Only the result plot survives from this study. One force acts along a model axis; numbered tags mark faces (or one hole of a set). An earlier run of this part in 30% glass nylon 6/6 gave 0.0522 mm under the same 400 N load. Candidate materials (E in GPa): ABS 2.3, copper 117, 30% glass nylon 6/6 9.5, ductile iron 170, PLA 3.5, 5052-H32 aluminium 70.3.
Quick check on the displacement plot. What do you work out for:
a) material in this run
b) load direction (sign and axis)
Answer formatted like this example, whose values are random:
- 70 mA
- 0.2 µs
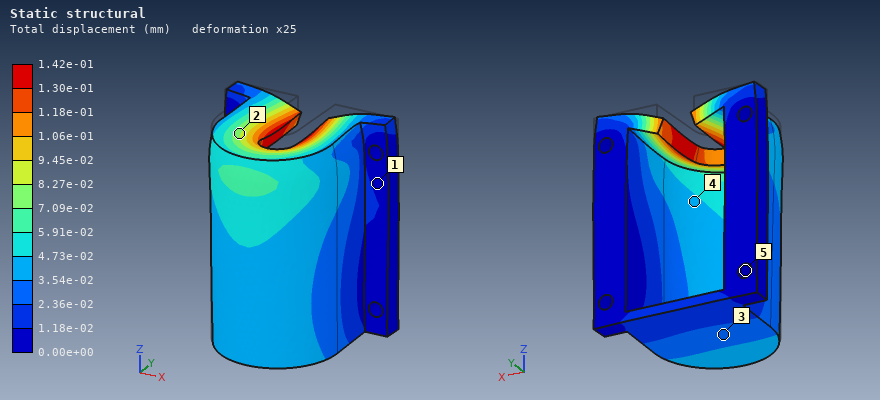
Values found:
- PLA
- -Z
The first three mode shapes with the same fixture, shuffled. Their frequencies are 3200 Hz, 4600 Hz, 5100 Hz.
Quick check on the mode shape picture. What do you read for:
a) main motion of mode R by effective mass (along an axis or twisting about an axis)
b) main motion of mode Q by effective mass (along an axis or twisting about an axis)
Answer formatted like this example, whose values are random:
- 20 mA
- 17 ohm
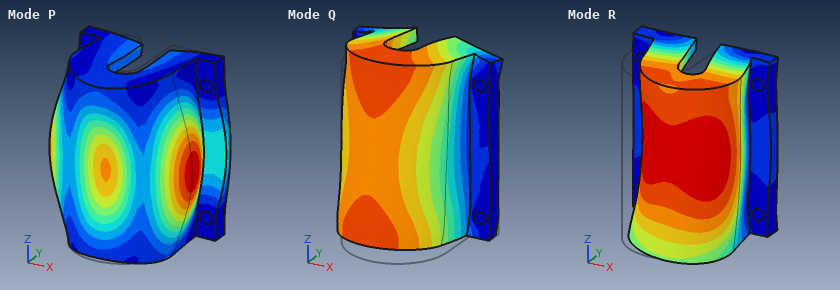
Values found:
- along X
- along Z
